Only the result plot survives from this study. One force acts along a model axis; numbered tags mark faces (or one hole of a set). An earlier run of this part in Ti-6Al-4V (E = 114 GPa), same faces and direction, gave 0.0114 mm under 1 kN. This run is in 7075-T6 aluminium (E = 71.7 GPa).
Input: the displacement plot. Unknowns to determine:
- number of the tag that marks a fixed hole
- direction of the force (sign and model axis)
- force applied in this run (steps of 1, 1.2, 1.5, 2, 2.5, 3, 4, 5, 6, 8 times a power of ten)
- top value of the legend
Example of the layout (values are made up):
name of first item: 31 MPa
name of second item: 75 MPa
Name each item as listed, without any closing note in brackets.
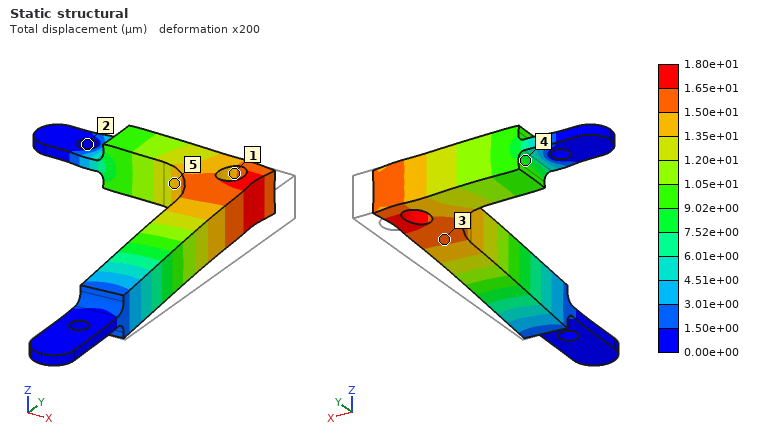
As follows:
number of the tag that marks a fixed hole: 2
direction of the force: -X
force applied in this run: 1 kN
top value of the legend: 1.80e+01 µm
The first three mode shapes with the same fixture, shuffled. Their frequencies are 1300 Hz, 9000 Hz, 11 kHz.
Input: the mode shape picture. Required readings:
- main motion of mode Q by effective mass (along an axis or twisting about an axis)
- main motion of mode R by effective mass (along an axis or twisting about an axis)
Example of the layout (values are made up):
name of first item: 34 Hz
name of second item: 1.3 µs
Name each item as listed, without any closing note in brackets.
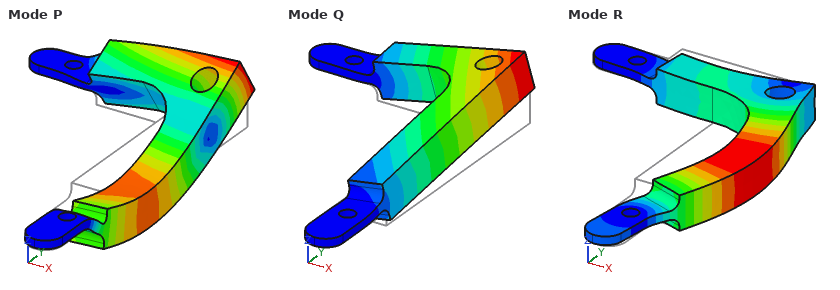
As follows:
main motion of mode Q by effective mass: along Z
main motion of mode R by effective mass: along X
